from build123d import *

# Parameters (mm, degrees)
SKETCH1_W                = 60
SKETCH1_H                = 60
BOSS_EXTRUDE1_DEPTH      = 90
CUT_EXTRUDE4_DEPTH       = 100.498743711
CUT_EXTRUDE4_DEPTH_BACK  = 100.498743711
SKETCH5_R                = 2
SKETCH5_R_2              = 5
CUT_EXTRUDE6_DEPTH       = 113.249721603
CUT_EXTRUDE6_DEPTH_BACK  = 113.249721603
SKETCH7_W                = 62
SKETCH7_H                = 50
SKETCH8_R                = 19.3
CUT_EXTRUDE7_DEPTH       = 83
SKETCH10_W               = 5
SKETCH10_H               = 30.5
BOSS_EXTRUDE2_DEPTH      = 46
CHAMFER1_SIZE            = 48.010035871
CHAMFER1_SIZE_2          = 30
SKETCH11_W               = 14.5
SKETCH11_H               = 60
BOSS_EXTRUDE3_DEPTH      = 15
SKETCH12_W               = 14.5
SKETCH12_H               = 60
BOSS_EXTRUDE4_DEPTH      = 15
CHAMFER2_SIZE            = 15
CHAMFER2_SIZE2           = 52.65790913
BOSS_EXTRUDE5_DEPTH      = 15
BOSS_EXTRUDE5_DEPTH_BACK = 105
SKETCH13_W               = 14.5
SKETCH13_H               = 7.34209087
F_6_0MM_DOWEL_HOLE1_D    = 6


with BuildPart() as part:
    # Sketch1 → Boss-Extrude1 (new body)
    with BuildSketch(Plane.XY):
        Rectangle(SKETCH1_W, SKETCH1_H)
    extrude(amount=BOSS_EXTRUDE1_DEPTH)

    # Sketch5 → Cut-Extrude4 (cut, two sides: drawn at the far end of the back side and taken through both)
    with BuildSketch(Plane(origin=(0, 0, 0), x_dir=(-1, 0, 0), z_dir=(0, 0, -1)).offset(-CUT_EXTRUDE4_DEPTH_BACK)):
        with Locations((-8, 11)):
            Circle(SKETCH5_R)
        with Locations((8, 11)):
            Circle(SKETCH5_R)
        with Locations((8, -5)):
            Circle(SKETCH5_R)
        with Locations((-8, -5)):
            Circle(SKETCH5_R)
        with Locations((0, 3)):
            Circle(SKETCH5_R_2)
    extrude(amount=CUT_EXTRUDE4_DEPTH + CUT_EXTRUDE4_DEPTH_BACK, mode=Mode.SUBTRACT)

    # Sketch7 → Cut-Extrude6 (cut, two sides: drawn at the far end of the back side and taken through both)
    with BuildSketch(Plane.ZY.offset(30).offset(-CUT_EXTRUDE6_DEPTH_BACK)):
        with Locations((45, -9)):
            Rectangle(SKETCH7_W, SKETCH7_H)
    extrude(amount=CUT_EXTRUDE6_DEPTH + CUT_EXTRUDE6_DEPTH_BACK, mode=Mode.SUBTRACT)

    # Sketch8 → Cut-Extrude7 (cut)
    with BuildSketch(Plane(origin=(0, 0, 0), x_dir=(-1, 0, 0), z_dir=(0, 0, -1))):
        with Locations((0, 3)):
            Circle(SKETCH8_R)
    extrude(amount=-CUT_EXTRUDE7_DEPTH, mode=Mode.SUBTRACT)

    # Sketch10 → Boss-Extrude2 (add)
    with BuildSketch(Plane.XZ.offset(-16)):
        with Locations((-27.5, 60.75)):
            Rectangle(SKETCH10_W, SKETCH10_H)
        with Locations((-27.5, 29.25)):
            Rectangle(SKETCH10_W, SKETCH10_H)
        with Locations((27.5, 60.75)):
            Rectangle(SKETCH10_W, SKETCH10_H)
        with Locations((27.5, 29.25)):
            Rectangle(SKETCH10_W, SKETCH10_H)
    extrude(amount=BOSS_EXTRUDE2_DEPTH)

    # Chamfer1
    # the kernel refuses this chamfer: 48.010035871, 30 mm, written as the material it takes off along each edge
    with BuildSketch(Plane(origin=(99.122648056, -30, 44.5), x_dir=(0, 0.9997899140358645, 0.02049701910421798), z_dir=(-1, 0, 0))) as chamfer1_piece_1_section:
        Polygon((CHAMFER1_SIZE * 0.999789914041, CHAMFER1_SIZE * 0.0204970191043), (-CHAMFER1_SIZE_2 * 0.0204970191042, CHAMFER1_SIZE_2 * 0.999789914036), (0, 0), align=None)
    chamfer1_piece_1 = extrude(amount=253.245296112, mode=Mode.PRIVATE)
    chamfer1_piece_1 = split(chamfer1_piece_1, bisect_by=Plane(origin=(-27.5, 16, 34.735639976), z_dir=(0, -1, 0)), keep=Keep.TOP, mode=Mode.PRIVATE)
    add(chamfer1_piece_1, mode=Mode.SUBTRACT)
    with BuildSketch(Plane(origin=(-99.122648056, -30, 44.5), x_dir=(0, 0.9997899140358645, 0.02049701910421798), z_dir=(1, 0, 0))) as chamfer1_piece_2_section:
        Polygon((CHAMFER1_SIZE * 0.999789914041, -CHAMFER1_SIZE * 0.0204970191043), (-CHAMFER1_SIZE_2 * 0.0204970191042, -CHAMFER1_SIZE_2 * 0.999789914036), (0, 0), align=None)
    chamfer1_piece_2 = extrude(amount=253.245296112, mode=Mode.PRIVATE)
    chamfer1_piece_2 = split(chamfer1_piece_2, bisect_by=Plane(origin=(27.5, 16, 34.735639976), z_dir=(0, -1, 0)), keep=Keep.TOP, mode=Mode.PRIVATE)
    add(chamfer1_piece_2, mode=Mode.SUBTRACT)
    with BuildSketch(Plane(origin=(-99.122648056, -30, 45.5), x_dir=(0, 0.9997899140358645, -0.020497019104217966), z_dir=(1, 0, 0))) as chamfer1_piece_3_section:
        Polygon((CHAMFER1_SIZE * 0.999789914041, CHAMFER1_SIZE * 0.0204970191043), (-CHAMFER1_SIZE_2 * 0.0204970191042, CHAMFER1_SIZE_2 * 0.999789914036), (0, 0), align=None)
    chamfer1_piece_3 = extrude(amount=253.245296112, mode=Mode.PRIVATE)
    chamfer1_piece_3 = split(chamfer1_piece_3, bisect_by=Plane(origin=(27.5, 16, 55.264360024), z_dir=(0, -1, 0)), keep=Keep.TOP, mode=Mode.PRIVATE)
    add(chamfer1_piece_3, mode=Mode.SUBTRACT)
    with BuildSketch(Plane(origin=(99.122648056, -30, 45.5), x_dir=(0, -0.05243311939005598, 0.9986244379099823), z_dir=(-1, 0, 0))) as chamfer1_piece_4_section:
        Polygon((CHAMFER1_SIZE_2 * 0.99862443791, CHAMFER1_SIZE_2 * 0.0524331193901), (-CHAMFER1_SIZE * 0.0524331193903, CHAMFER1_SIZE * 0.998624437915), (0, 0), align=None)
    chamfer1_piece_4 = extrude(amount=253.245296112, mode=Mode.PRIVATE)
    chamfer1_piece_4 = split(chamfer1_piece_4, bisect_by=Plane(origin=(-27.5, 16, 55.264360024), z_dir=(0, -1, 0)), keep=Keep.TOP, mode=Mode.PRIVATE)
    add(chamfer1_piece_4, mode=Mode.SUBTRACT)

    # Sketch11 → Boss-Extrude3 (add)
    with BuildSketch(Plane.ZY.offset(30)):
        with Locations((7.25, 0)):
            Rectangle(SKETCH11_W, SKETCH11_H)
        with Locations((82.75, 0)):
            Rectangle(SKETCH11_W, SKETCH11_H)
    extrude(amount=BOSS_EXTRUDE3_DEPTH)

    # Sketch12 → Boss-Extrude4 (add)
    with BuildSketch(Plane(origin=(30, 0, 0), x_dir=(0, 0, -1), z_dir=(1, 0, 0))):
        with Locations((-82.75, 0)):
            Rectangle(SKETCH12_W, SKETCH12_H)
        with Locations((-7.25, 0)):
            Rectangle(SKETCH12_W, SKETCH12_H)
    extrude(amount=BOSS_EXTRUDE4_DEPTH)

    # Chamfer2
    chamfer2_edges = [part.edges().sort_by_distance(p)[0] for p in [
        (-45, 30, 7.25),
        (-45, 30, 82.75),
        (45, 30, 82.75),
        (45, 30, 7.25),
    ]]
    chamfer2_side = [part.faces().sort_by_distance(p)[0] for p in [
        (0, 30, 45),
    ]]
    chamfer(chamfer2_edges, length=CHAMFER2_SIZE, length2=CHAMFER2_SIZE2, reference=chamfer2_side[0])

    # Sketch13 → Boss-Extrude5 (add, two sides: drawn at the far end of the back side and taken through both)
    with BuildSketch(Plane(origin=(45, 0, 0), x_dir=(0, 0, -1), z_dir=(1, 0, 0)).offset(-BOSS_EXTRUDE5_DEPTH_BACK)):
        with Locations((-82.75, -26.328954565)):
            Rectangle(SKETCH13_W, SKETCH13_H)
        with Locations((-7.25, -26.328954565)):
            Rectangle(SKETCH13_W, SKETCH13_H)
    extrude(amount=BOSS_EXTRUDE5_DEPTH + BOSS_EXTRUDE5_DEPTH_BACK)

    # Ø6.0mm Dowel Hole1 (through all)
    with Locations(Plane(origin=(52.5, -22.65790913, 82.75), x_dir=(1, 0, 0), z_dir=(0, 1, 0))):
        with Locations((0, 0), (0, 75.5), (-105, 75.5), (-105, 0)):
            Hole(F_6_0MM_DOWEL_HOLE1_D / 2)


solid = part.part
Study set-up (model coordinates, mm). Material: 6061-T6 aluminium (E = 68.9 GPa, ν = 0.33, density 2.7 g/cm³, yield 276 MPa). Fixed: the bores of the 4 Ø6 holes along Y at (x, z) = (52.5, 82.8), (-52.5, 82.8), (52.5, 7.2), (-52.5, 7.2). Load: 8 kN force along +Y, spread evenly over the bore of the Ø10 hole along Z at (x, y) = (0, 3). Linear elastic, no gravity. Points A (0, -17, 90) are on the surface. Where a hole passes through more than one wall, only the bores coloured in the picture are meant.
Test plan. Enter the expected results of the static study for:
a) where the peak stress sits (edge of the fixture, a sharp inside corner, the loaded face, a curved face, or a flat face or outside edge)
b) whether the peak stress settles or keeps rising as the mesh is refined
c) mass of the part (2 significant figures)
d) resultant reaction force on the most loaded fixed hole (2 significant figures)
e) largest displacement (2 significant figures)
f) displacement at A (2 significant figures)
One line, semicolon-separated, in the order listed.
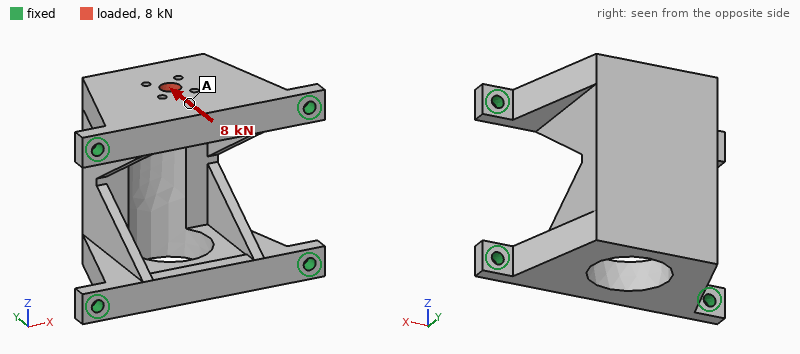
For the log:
edge of the fixture; keeps rising; 460 g; 5.1 kN; 61 µm; 54 µm
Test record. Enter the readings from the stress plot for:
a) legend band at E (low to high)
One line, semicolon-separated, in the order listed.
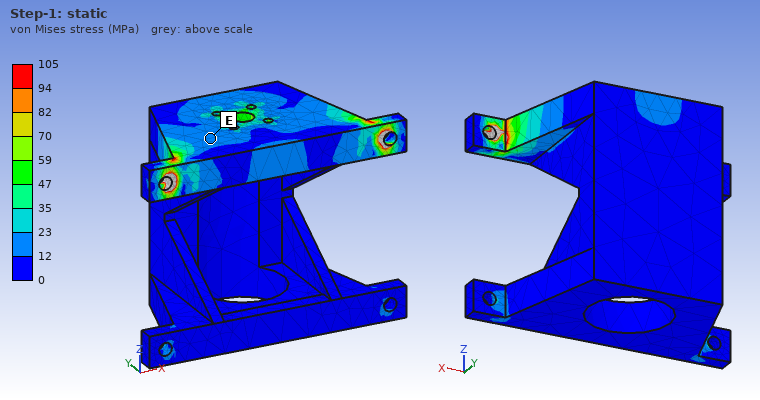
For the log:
12 to 23 MPa
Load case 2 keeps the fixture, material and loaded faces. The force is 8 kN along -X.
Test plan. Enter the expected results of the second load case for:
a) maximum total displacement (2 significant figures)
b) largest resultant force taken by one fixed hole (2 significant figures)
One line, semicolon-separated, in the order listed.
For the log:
34 µm; 4.3 kN
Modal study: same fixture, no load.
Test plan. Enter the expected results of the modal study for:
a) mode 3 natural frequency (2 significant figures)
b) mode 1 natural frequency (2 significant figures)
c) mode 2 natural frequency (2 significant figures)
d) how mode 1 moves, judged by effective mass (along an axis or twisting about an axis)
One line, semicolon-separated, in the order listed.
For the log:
4600 Hz; 2300 Hz; 4500 Hz; along Z
